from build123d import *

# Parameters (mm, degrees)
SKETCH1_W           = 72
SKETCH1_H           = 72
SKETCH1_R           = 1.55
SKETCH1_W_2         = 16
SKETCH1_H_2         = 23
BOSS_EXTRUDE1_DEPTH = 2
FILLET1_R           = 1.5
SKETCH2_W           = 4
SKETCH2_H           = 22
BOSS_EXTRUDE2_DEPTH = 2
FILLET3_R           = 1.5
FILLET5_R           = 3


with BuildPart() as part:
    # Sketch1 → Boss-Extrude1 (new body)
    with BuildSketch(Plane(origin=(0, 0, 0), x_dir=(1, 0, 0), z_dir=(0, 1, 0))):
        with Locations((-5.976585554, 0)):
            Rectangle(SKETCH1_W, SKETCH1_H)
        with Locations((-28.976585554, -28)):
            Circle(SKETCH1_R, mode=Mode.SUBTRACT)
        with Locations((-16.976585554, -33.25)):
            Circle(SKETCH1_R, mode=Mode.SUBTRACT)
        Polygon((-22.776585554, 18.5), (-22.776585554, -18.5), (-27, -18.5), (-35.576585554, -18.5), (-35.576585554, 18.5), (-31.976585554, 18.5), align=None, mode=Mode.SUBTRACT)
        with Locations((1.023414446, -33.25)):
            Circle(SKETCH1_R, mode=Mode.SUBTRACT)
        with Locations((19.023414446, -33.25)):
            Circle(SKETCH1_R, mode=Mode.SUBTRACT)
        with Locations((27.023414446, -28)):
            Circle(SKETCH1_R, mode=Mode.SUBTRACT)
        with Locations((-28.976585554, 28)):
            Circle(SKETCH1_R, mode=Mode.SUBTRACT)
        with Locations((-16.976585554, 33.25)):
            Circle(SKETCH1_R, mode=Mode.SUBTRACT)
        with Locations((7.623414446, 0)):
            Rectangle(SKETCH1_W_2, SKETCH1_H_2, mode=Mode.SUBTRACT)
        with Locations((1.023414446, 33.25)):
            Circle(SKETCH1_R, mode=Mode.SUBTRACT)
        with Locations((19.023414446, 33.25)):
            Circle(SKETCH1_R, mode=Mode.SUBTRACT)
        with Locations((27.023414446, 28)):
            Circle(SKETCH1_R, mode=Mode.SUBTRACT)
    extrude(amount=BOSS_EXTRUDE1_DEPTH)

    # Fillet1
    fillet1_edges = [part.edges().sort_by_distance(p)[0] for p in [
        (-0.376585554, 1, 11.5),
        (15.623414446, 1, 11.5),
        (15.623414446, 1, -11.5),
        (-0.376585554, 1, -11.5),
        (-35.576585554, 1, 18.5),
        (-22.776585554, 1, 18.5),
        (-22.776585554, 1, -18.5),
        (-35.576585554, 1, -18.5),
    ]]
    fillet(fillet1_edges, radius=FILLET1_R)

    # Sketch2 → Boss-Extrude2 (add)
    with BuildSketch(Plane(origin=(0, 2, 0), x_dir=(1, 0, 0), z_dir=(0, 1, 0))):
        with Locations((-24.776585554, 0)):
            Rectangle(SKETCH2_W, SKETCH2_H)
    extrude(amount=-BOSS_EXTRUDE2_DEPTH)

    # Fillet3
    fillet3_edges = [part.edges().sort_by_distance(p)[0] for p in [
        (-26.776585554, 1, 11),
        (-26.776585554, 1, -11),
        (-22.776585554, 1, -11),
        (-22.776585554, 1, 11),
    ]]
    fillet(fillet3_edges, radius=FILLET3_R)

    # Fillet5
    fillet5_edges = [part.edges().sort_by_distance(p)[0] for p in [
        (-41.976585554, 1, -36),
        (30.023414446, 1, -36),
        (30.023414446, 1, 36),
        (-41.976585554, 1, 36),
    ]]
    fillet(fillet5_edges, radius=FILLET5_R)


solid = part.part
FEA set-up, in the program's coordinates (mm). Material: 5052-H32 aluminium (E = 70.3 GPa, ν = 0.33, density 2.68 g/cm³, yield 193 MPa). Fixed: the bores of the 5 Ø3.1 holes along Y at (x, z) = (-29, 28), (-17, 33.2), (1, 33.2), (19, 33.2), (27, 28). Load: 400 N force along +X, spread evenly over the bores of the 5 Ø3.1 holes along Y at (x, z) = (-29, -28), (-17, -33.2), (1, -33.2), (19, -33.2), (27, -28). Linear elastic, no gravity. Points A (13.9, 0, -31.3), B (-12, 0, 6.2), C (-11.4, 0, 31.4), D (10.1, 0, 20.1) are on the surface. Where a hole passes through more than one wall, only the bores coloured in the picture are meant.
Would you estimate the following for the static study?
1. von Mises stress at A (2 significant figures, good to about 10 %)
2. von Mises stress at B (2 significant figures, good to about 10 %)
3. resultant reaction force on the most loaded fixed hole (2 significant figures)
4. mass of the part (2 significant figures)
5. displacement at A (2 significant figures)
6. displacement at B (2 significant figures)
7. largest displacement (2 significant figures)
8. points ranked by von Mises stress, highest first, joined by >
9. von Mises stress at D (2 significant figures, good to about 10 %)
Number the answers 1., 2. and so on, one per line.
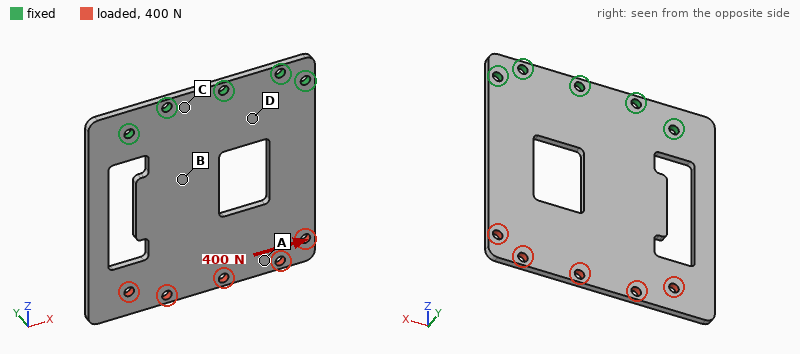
1. 6.5 MPa
2. 16 MPa
3. 370 N
4. 23 g
5. 32 µm
6. 8.9 µm
7. 36 µm
8. B > D > A > C
9. 12 MPa
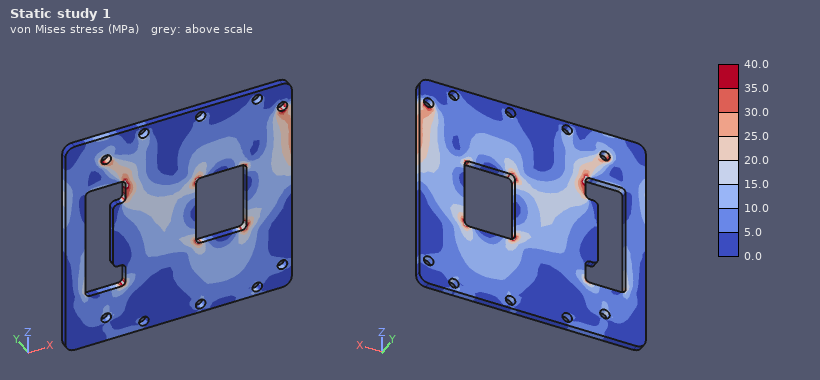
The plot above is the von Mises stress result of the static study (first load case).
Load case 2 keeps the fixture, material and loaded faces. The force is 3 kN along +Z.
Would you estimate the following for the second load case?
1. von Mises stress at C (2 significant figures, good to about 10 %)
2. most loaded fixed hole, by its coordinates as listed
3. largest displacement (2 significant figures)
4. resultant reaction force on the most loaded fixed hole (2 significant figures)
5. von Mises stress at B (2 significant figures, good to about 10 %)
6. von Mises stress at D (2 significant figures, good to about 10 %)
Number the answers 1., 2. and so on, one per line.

1. 14 MPa
2. (27, 28)
3. 38 µm
4. 740 N
5. 30 MPa
6. 8.5 MPa
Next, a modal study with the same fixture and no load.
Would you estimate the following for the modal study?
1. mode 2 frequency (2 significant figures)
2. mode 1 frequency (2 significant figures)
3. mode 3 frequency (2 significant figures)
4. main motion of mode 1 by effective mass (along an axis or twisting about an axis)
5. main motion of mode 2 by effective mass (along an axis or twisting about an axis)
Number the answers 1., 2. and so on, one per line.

1. 830 Hz
2. 350 Hz
3. 2200 Hz
4. along Y
5. twisting about Z
